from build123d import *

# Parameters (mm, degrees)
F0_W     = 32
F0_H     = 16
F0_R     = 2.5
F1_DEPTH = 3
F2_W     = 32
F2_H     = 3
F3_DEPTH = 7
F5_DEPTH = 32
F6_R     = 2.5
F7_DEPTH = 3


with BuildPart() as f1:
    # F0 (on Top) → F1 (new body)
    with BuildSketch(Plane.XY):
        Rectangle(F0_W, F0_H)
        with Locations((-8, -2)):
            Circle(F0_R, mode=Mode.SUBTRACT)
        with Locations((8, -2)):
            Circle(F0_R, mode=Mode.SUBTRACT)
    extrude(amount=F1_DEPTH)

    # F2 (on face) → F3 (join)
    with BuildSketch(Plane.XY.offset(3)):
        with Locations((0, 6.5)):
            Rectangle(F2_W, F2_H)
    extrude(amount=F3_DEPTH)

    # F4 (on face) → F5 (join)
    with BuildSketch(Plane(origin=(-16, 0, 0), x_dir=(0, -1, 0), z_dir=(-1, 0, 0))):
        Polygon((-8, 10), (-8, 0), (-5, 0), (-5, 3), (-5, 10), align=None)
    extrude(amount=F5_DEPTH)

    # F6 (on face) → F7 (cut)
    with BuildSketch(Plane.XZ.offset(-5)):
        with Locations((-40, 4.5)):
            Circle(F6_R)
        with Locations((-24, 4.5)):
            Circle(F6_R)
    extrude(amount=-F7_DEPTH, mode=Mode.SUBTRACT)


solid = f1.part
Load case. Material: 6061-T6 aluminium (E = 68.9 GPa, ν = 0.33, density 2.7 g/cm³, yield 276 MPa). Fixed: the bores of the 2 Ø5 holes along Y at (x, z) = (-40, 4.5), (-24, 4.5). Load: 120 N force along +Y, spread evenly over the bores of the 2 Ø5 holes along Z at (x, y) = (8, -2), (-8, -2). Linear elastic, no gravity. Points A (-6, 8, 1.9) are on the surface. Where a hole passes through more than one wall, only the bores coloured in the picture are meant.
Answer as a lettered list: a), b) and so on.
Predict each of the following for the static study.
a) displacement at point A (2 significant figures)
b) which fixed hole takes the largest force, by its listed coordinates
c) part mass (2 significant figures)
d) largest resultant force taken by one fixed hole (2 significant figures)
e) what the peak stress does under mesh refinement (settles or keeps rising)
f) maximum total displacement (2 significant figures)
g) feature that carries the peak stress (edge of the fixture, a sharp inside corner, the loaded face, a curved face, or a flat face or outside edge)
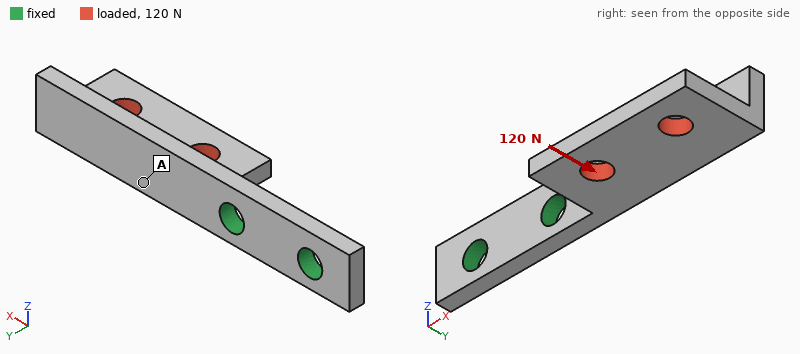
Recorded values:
a) 0.16 mm
b) (-24, 4.5)
c) 7.9 g
d) 120 N
e) keeps rising
f) 0.49 mm
g) edge of the fixture
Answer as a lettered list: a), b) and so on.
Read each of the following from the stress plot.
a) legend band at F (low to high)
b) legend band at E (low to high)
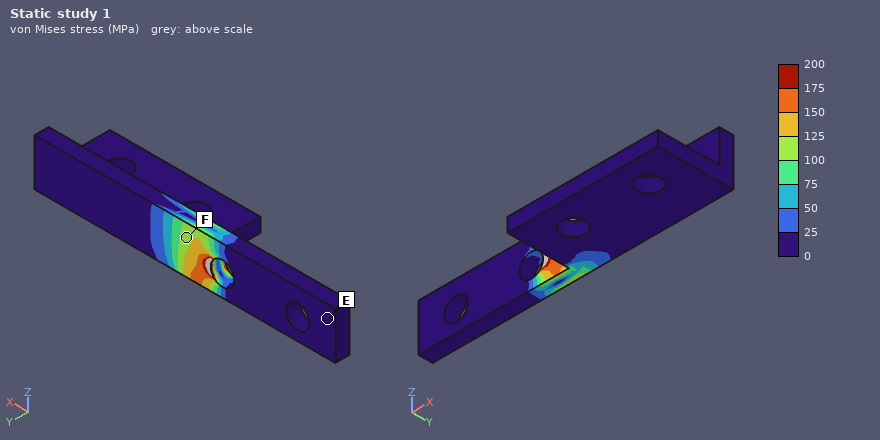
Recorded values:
a) 100 to 125 MPa
b) 0 to 25 MPa
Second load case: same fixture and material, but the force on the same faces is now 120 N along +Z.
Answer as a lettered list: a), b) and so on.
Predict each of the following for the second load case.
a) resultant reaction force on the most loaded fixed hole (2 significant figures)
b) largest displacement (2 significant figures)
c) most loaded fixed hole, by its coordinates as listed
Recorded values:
a) 160 N
b) 0.19 mm
c) (-24, 4.5)
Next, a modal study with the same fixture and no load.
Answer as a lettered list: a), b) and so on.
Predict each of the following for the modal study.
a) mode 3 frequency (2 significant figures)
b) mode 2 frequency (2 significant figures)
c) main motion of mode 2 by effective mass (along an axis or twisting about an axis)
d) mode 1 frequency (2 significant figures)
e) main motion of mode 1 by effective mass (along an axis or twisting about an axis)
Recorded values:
a) 5200 Hz
b) 2800 Hz
c) along Z
d) 1300 Hz
e) along Y
